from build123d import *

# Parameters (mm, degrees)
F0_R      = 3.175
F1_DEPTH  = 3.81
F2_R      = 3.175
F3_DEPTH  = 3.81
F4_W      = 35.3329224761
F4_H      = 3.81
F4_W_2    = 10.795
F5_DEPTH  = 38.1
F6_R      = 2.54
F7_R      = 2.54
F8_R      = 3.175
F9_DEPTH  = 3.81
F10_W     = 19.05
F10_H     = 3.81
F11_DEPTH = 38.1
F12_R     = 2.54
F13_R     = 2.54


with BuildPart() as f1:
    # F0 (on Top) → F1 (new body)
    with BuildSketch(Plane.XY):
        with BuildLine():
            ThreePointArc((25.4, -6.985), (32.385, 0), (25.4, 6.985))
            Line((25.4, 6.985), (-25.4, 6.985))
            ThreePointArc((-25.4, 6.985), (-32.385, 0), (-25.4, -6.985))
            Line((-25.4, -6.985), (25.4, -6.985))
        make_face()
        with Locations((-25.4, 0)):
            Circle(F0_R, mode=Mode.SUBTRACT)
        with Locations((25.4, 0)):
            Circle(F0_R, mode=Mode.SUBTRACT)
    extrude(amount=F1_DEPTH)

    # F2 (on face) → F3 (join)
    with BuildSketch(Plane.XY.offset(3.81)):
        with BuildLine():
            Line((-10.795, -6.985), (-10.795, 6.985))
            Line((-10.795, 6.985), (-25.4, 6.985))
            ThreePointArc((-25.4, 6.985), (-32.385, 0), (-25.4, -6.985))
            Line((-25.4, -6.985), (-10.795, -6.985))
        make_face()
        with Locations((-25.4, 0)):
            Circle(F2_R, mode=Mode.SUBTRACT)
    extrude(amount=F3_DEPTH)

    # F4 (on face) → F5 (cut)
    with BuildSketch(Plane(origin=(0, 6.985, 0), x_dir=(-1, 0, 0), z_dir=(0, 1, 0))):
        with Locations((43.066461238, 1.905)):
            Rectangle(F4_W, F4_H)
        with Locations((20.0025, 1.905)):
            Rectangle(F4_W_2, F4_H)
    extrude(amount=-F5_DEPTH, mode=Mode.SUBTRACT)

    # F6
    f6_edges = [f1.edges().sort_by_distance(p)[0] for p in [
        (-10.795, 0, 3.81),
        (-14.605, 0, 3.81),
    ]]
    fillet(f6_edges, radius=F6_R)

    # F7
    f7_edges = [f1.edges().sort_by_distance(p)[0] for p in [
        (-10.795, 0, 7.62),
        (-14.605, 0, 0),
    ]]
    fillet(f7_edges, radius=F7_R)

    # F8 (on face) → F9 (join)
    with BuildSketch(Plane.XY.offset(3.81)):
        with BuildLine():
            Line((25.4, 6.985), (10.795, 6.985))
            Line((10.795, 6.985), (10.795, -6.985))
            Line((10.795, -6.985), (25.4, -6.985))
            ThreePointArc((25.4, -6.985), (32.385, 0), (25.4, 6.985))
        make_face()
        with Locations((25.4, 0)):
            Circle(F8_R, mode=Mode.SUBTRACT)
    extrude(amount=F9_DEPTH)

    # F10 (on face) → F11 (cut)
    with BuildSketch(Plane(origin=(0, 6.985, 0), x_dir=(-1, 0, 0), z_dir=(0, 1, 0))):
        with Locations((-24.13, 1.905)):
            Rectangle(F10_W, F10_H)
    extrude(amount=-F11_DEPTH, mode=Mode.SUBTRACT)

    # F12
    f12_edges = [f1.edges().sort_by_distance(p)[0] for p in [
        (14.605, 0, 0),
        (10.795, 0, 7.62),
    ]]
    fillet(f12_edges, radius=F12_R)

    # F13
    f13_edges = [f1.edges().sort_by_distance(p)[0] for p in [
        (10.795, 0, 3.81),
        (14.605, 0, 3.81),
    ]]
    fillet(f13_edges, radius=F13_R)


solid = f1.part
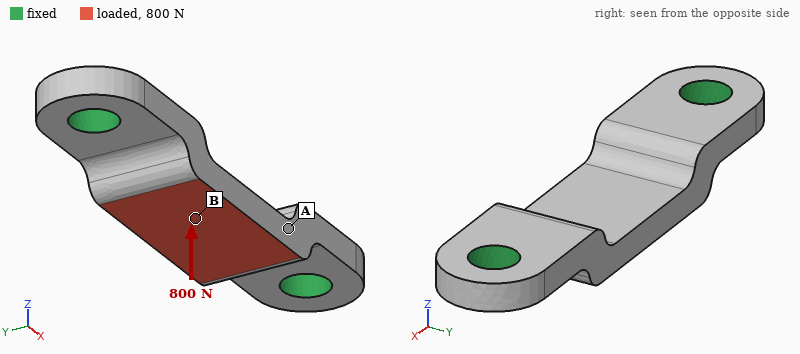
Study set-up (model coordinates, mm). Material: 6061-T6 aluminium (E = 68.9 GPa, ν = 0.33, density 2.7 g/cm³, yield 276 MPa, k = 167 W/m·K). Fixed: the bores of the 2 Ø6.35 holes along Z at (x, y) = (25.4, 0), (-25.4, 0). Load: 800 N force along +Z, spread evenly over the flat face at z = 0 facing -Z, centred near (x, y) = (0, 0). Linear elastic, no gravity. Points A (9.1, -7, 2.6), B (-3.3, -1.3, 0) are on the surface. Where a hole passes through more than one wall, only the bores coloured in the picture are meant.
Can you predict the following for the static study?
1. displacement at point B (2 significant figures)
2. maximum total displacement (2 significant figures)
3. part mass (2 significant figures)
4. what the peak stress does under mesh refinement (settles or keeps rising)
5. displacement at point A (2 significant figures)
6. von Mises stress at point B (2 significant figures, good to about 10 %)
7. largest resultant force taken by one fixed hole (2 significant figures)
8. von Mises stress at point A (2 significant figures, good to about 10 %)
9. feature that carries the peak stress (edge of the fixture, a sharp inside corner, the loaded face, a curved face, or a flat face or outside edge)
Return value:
30 µm
33 µm
9.3 g
keeps rising
22 µm
43 MPa
950 N
20 MPa
edge of the fixture
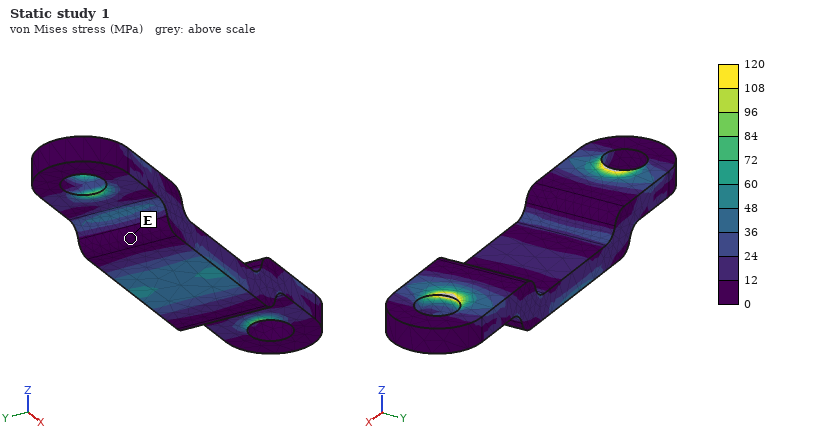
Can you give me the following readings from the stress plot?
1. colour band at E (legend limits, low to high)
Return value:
0 to 12 MPa
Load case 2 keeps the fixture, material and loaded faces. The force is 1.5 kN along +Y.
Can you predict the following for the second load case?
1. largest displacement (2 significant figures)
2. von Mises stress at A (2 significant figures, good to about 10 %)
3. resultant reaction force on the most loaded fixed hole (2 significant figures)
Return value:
75 µm
35 MPa
750 N
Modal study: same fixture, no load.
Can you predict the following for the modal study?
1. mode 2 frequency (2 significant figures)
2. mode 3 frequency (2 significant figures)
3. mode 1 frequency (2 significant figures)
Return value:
13 kHz
21 kHz
13 kHz
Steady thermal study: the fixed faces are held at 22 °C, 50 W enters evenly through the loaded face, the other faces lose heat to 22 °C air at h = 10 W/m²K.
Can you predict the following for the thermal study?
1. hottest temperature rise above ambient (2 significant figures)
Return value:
49 K
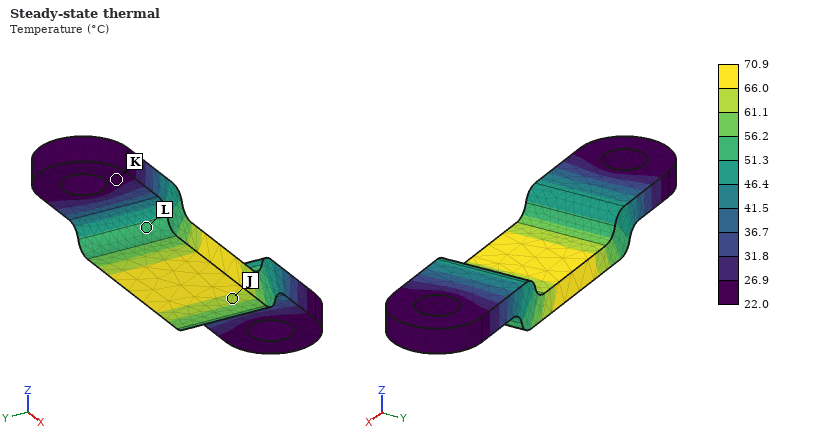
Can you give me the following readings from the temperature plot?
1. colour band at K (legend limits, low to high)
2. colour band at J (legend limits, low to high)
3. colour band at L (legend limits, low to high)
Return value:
22.0 to 26.9 °C
61.1 to 66.0 °C
51.3 to 56.2 °C
